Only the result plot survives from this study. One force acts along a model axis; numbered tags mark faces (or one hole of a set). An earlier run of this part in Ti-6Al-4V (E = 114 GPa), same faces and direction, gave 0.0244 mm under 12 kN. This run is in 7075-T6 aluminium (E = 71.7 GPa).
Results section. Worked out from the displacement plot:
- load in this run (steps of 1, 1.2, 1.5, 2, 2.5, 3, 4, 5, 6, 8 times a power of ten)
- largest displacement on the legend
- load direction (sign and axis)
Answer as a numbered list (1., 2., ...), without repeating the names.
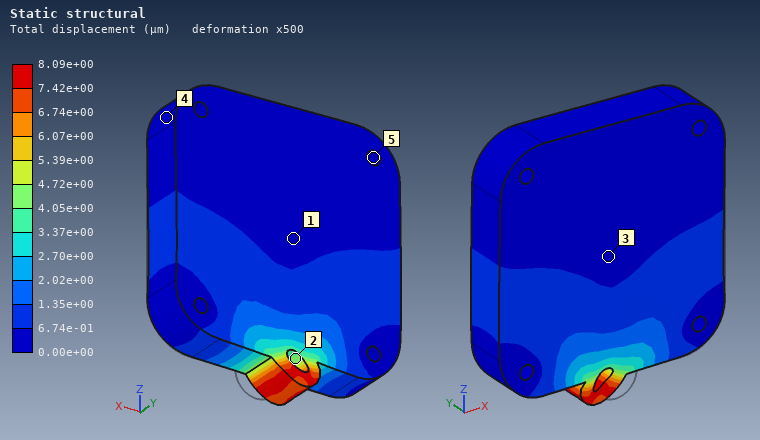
1. 2.5 kN
2. 8.09e+00 µm
3. -X
